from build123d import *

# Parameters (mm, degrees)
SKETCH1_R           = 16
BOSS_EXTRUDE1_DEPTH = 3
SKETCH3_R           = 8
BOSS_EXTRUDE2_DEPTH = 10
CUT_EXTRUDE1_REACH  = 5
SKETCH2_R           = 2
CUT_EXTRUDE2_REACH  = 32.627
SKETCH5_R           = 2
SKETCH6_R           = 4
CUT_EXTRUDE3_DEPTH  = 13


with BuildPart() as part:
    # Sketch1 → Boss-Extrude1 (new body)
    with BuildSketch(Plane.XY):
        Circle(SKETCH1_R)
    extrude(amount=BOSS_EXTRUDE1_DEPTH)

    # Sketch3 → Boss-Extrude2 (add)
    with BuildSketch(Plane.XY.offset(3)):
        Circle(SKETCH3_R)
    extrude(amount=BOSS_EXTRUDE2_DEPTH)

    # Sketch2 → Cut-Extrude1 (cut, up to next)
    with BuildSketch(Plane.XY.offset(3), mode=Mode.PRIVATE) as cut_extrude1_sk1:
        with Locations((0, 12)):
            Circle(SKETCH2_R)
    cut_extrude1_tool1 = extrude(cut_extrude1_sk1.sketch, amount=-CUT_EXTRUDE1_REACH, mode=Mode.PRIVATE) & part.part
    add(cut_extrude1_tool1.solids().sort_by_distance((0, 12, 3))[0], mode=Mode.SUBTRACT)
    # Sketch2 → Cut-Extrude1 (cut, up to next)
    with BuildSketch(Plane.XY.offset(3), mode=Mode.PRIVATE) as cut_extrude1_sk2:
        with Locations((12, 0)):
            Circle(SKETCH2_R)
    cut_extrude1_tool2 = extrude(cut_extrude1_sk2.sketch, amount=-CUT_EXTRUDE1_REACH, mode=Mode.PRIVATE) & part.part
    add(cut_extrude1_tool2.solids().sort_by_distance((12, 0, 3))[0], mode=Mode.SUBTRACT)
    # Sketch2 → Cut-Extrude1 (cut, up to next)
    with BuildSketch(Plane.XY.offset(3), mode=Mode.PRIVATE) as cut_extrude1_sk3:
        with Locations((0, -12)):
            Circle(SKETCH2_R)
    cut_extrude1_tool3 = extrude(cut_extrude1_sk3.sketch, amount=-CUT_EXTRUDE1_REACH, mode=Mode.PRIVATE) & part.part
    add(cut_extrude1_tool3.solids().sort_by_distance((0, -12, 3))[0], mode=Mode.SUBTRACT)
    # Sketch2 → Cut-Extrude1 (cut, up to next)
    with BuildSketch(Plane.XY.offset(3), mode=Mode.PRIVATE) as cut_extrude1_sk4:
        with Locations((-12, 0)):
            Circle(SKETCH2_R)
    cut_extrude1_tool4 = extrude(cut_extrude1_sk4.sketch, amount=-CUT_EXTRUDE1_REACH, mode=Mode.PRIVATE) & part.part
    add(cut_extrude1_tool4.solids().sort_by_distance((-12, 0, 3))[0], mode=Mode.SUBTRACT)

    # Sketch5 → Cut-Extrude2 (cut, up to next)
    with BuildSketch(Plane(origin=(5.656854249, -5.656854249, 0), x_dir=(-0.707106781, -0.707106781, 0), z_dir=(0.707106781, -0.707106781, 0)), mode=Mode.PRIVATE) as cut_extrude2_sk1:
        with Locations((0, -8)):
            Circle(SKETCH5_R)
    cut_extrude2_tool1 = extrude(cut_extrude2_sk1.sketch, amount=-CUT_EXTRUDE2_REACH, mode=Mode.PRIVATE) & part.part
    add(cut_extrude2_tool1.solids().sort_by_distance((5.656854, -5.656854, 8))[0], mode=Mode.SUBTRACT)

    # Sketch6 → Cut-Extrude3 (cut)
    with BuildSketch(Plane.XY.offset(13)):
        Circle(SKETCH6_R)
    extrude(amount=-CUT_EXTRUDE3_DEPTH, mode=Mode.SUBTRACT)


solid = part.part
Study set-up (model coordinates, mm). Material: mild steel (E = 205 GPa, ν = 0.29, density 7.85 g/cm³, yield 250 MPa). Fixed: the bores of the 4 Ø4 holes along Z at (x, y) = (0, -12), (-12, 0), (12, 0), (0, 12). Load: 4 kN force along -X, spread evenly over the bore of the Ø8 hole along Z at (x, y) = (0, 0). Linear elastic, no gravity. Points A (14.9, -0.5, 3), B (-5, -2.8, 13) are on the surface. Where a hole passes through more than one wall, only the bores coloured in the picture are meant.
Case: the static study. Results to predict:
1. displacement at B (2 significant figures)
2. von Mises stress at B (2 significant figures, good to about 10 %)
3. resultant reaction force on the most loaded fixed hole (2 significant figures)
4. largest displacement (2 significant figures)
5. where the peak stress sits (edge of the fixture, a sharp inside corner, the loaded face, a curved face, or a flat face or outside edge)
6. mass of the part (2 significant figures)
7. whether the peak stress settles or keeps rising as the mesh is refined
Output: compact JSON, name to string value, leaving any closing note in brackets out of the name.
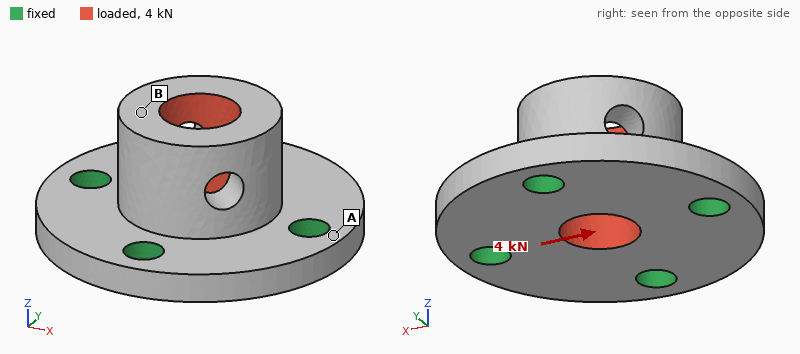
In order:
{"displacement at B": "8.4 µm", "von Mises stress at B": "24 MPa", "resultant reaction force on the most loaded fixed hole": "1.6 kN", "largest displacement": "8.9 µm", "where the peak stress sits": "edge of the fixture", "mass of the part": "28 g", "whether the peak stress settles or keeps rising as the mesh is refined": "keeps rising"}
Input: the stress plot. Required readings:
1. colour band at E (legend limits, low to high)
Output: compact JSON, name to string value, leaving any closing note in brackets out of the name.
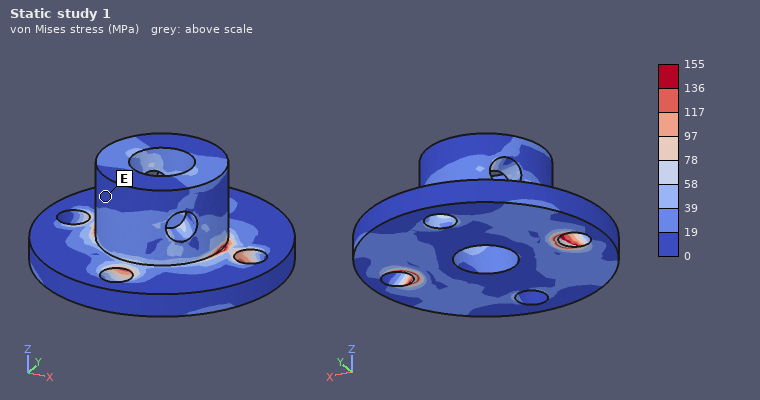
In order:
{"colour band at E": "0 to 19 MPa"}
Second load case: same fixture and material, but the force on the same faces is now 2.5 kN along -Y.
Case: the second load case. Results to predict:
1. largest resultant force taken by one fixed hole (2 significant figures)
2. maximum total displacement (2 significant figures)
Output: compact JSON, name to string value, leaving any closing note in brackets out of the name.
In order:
{"largest resultant force taken by one fixed hole": "1000 N", "maximum total displacement": "5.6 µm"}
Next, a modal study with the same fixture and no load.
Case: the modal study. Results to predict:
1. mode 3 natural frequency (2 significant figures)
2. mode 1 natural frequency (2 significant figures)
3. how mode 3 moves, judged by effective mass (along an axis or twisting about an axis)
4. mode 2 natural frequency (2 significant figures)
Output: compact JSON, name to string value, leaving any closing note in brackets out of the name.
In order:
{"mode 3 natural frequency": "39 kHz", "mode 1 natural frequency": "31 kHz", "how mode 3 moves, judged by effective mass": "along Z", "mode 2 natural frequency": "32 kHz"}
